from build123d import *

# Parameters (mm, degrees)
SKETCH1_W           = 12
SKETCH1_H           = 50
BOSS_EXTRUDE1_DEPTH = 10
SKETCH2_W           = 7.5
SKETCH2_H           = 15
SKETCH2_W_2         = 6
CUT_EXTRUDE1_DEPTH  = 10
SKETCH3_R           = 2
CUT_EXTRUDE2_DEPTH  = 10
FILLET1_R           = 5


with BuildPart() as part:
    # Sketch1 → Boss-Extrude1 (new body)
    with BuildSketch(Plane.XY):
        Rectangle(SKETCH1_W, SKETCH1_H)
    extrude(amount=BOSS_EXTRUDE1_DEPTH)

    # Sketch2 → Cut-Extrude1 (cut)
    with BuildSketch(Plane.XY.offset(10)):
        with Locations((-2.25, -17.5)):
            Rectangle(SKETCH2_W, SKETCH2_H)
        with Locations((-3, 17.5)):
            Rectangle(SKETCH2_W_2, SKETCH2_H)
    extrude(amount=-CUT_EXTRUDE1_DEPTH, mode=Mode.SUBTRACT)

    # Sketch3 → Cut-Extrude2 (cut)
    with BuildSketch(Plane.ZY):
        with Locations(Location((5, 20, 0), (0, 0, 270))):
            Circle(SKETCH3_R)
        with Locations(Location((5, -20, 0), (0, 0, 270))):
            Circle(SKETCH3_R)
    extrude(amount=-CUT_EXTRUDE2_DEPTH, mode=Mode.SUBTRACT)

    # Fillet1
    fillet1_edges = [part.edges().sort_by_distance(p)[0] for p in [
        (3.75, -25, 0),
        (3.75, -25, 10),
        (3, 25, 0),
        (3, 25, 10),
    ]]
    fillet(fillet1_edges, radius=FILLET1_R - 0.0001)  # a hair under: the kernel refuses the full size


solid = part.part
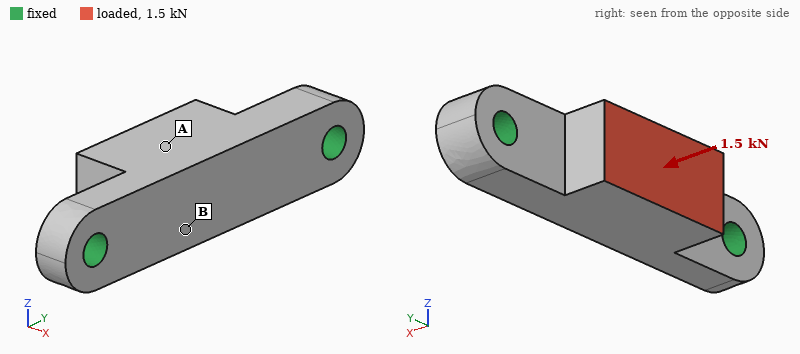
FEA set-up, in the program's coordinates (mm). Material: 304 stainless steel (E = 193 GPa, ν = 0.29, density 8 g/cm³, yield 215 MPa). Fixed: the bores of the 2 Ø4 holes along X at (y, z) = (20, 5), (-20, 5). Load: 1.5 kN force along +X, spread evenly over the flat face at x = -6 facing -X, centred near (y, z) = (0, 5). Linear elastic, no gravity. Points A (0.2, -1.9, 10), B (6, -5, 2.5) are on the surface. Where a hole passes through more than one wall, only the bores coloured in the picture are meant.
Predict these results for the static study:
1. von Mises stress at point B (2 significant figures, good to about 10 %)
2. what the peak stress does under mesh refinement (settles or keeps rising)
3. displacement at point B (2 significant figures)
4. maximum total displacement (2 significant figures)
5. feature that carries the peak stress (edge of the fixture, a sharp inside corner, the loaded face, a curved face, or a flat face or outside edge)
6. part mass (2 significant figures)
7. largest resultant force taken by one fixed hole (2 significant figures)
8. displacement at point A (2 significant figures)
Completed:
32 MPa
keeps rising
8.2 µm
8.6 µm
edge of the fixture
30 g
840 N
8.2 µm
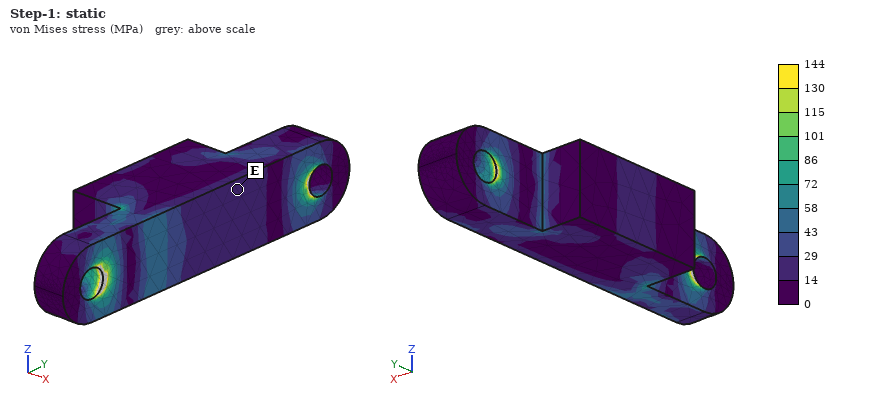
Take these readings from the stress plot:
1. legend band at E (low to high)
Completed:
14 to 29 MPa
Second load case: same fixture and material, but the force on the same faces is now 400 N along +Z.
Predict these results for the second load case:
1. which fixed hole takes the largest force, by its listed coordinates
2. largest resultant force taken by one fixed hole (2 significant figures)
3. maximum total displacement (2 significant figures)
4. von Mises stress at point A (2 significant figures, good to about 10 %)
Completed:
(20, 5)
210 N
10 µm
8.8 MPa
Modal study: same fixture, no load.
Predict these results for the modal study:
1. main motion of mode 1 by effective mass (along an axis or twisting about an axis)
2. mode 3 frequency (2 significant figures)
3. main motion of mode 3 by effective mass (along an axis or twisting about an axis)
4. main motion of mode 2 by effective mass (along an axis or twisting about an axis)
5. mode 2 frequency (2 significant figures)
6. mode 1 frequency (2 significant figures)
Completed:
along Z
23 kHz
along Z
along X
15 kHz
12 kHz
